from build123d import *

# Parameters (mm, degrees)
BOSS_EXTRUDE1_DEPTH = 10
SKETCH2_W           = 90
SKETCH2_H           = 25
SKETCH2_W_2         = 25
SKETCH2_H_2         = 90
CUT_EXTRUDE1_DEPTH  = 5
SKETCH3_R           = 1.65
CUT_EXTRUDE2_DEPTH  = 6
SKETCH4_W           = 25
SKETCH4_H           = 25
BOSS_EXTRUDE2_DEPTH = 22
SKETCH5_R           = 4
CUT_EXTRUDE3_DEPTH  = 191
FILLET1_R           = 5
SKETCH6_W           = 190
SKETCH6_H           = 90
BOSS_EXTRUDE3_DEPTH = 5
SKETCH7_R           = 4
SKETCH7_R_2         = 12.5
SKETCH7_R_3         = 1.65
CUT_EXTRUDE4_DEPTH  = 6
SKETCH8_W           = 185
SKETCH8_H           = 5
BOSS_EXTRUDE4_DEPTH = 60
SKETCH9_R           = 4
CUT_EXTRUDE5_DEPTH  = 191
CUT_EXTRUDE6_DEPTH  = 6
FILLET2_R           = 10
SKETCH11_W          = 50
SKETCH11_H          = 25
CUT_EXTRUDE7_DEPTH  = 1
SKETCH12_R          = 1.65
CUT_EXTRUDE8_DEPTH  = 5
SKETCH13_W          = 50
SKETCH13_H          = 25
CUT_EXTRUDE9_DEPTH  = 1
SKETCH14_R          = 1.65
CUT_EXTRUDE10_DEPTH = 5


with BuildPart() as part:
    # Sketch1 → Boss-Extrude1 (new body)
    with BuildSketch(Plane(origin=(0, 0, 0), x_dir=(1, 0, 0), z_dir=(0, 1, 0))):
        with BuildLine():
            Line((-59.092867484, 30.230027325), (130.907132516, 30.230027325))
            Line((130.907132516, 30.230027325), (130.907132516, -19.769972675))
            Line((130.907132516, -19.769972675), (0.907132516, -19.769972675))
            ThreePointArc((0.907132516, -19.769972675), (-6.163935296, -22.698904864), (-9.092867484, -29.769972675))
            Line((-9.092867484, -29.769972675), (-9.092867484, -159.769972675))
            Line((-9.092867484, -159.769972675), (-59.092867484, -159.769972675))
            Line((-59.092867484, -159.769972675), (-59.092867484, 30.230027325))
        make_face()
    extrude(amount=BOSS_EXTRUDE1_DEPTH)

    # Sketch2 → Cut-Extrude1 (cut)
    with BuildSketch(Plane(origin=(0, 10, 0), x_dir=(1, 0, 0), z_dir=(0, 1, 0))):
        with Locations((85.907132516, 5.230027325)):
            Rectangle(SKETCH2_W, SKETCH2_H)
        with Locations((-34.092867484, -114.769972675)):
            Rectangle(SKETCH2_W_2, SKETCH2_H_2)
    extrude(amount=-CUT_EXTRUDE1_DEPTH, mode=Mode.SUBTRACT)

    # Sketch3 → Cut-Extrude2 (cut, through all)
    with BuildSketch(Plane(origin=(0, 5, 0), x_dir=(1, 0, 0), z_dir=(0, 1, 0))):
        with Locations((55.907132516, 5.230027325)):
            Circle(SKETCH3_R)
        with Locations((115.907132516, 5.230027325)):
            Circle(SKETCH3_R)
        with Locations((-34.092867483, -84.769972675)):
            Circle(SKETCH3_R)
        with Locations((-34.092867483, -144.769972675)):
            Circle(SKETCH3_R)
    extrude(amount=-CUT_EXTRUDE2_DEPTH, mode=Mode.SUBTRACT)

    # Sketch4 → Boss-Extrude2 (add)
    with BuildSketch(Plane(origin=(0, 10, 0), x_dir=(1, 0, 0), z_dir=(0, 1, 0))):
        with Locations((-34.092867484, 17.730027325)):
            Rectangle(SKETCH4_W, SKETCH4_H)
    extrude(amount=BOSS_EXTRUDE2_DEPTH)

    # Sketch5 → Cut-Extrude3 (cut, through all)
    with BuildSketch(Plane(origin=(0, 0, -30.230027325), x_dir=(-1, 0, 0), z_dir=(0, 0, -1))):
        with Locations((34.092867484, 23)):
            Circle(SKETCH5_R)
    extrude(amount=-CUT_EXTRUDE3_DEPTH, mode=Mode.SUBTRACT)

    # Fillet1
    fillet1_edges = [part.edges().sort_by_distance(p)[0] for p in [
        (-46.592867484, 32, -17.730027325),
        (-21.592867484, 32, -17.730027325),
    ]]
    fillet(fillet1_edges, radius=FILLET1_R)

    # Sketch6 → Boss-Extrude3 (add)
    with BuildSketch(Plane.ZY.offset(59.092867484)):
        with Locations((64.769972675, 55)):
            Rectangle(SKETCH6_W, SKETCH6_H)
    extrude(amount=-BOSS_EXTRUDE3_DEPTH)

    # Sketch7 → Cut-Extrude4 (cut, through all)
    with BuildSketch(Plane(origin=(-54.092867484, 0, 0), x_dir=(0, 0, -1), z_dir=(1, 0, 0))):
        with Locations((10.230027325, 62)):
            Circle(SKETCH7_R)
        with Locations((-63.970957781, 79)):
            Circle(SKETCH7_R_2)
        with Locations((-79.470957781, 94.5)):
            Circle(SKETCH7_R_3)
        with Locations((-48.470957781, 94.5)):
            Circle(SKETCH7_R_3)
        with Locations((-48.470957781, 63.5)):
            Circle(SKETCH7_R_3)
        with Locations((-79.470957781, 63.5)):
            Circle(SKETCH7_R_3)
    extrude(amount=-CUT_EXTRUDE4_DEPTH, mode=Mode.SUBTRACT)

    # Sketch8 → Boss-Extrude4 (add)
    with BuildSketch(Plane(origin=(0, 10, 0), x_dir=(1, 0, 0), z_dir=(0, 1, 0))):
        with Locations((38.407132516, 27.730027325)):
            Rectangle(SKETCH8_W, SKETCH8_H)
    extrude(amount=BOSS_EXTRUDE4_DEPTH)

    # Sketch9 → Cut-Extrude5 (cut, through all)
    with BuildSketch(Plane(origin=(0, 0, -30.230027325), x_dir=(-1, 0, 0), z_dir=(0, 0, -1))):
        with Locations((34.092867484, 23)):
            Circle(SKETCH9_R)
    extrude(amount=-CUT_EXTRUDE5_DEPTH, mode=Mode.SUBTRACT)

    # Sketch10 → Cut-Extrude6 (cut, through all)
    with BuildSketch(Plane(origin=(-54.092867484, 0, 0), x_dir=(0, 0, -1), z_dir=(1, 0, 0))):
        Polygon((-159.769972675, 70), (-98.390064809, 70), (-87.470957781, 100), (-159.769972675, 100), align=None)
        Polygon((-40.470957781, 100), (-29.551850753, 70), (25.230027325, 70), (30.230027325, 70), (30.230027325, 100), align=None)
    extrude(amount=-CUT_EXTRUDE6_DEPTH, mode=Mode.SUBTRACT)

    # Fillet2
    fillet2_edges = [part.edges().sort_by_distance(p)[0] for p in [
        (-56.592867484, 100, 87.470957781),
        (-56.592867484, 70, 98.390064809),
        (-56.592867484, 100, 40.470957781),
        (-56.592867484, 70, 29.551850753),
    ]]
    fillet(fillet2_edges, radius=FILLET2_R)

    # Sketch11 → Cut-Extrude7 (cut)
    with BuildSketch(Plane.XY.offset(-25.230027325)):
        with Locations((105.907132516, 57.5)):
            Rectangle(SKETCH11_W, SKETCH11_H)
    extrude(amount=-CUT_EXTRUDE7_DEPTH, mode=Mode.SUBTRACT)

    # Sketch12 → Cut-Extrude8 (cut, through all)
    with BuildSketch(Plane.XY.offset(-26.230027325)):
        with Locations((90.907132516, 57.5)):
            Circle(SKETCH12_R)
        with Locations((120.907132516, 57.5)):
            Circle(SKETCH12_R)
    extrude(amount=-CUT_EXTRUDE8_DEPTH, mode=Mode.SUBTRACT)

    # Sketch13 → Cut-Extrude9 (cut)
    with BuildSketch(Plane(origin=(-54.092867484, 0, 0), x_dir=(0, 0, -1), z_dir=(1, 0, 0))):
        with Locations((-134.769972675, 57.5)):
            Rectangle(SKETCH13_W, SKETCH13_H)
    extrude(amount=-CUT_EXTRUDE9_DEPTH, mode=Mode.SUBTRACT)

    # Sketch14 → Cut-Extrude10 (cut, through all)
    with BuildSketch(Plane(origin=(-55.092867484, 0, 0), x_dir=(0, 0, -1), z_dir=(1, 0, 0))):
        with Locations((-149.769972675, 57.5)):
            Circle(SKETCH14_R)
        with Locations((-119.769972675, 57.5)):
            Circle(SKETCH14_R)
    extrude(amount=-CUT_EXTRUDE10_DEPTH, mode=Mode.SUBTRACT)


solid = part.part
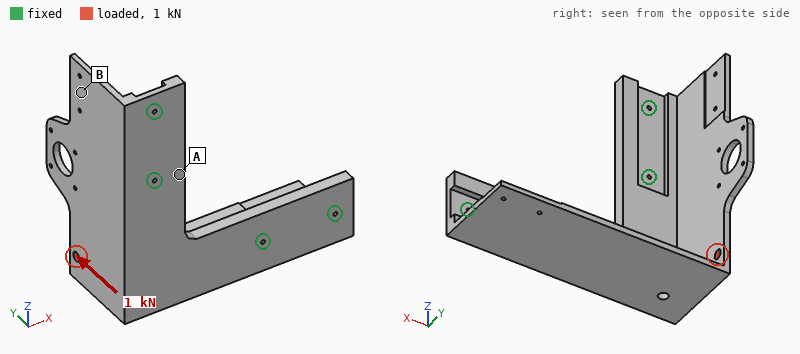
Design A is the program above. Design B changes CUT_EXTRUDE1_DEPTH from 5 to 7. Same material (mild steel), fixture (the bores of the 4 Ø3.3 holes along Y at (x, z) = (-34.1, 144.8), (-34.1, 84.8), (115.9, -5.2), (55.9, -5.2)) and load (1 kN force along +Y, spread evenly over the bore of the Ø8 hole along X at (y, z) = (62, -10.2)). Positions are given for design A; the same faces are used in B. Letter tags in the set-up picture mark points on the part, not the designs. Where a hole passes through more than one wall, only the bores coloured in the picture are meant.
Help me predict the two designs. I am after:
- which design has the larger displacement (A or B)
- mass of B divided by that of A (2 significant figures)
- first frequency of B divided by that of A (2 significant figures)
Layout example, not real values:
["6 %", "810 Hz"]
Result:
["B", "0.97", "0.76"]
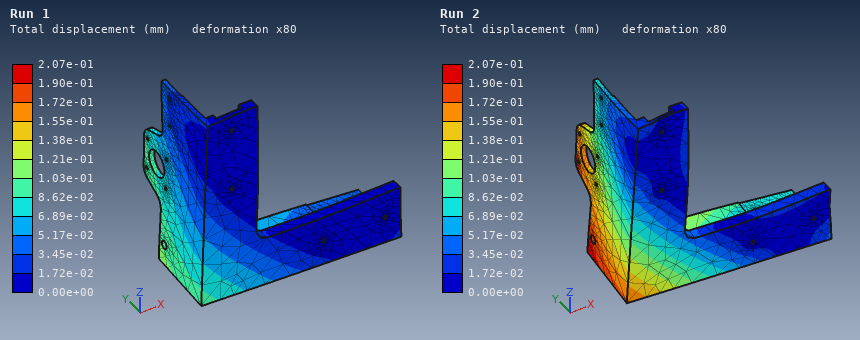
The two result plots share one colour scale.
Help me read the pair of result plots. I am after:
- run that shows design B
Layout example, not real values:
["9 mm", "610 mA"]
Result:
["Run 2"]
